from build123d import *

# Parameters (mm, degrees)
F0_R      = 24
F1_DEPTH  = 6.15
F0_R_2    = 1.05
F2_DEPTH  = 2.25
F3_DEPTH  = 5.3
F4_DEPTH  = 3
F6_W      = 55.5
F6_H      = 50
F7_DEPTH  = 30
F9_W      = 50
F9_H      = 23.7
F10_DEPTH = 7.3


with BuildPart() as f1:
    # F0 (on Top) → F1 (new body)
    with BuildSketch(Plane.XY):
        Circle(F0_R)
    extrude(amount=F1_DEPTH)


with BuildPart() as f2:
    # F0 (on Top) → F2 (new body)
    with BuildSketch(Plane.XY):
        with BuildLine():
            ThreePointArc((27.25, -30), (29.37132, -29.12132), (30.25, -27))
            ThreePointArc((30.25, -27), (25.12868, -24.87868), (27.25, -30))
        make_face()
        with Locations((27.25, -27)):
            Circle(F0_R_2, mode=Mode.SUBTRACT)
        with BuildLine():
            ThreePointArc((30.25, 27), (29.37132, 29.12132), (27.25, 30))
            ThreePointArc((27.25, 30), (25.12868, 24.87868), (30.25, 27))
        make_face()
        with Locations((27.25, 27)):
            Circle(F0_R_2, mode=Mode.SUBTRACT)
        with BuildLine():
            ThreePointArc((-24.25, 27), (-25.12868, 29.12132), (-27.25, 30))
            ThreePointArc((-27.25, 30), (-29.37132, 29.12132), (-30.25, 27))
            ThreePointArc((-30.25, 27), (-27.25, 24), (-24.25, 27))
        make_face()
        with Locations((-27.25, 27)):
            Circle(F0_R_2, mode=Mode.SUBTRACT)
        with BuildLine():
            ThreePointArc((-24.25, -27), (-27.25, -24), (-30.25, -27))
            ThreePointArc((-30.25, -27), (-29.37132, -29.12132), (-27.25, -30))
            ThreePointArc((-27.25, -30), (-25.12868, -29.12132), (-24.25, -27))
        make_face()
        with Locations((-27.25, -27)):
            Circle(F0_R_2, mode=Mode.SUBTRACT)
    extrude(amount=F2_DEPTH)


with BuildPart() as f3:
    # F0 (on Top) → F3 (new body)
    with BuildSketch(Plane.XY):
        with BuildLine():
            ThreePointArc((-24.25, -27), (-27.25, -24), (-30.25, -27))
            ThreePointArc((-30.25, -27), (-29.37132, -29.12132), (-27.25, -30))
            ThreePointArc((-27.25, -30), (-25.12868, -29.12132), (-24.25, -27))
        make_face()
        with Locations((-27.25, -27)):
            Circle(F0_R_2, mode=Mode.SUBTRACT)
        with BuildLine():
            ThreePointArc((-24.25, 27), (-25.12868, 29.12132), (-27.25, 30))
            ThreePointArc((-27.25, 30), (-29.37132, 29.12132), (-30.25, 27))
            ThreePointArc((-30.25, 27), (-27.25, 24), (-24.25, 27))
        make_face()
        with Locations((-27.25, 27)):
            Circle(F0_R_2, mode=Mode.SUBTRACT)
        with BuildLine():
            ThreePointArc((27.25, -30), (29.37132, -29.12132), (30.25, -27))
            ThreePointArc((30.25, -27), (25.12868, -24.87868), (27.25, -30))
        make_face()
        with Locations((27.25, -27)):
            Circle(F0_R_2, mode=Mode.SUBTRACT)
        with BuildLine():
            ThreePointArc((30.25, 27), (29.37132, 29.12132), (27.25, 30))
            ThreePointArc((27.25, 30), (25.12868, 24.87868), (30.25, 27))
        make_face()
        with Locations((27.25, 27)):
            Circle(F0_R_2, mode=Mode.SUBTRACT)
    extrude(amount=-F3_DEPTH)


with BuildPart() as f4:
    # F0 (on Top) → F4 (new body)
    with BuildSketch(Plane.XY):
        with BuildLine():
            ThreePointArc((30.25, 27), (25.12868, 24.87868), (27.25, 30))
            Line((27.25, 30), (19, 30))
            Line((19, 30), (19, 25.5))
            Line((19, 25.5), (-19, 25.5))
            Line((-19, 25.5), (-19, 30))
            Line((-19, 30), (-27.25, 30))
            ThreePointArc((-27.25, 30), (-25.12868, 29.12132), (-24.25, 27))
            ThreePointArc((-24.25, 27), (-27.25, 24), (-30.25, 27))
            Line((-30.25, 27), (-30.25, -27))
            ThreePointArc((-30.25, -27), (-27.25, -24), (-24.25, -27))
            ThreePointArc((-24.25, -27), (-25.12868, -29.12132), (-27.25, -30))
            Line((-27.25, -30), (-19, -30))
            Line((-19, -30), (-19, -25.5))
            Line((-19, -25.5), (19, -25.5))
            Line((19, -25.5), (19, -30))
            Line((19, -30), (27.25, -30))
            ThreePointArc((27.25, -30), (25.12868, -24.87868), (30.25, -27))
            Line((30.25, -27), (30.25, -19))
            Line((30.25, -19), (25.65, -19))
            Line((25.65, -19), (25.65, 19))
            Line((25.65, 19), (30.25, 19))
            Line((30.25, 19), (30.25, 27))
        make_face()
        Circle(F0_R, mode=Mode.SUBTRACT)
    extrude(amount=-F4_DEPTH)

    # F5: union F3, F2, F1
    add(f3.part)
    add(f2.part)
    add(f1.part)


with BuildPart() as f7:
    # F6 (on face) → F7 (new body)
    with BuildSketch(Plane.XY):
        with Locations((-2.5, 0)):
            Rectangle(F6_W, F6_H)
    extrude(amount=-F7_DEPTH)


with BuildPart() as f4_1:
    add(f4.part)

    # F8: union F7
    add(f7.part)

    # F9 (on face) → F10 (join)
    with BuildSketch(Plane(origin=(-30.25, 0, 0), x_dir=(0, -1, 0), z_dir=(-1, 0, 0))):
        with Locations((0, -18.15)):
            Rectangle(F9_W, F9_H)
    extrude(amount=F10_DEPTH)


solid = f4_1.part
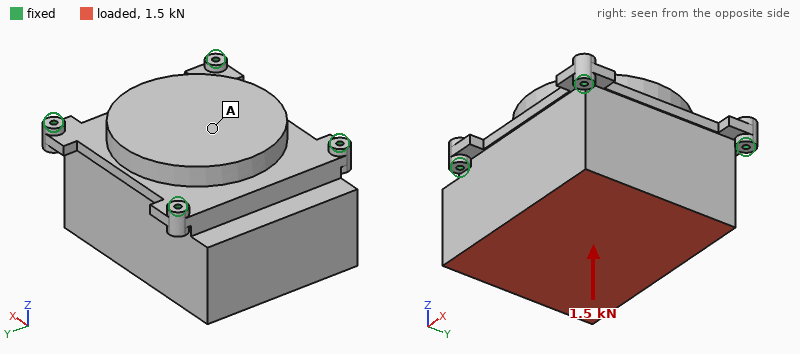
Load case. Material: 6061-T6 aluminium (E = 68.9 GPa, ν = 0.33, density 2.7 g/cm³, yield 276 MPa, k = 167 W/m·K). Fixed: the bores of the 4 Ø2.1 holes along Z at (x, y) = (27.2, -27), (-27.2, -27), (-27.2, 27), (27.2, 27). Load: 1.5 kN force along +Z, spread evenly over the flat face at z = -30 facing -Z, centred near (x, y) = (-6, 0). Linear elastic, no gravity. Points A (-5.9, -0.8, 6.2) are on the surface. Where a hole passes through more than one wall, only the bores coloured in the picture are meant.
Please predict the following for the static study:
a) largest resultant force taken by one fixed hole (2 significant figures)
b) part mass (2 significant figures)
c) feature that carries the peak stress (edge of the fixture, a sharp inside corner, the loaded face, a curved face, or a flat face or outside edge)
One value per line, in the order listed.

500 N
280 g
a flat face or outside edge
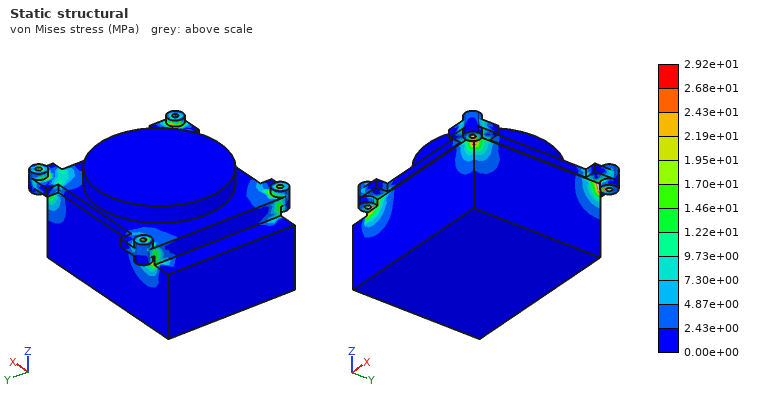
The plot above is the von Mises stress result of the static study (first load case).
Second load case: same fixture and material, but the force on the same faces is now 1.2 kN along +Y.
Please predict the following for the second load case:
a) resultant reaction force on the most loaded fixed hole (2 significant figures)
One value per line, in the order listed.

610 N
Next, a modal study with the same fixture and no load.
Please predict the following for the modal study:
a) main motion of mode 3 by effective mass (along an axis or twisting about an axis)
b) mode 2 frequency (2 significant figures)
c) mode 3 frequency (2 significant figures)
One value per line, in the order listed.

along Y
6700 Hz
7100 Hz
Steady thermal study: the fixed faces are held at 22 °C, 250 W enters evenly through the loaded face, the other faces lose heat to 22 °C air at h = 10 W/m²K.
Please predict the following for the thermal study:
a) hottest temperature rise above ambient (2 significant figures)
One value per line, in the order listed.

78 K
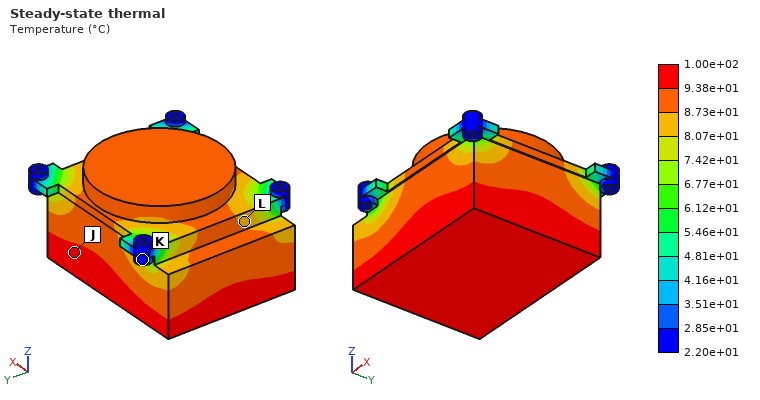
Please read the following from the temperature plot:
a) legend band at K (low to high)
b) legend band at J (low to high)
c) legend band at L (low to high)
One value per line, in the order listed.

2.20e+01 to 2.85e+01 °C
9.38e+01 to 1.00e+02 °C
8.07e+01 to 8.73e+01 °C
